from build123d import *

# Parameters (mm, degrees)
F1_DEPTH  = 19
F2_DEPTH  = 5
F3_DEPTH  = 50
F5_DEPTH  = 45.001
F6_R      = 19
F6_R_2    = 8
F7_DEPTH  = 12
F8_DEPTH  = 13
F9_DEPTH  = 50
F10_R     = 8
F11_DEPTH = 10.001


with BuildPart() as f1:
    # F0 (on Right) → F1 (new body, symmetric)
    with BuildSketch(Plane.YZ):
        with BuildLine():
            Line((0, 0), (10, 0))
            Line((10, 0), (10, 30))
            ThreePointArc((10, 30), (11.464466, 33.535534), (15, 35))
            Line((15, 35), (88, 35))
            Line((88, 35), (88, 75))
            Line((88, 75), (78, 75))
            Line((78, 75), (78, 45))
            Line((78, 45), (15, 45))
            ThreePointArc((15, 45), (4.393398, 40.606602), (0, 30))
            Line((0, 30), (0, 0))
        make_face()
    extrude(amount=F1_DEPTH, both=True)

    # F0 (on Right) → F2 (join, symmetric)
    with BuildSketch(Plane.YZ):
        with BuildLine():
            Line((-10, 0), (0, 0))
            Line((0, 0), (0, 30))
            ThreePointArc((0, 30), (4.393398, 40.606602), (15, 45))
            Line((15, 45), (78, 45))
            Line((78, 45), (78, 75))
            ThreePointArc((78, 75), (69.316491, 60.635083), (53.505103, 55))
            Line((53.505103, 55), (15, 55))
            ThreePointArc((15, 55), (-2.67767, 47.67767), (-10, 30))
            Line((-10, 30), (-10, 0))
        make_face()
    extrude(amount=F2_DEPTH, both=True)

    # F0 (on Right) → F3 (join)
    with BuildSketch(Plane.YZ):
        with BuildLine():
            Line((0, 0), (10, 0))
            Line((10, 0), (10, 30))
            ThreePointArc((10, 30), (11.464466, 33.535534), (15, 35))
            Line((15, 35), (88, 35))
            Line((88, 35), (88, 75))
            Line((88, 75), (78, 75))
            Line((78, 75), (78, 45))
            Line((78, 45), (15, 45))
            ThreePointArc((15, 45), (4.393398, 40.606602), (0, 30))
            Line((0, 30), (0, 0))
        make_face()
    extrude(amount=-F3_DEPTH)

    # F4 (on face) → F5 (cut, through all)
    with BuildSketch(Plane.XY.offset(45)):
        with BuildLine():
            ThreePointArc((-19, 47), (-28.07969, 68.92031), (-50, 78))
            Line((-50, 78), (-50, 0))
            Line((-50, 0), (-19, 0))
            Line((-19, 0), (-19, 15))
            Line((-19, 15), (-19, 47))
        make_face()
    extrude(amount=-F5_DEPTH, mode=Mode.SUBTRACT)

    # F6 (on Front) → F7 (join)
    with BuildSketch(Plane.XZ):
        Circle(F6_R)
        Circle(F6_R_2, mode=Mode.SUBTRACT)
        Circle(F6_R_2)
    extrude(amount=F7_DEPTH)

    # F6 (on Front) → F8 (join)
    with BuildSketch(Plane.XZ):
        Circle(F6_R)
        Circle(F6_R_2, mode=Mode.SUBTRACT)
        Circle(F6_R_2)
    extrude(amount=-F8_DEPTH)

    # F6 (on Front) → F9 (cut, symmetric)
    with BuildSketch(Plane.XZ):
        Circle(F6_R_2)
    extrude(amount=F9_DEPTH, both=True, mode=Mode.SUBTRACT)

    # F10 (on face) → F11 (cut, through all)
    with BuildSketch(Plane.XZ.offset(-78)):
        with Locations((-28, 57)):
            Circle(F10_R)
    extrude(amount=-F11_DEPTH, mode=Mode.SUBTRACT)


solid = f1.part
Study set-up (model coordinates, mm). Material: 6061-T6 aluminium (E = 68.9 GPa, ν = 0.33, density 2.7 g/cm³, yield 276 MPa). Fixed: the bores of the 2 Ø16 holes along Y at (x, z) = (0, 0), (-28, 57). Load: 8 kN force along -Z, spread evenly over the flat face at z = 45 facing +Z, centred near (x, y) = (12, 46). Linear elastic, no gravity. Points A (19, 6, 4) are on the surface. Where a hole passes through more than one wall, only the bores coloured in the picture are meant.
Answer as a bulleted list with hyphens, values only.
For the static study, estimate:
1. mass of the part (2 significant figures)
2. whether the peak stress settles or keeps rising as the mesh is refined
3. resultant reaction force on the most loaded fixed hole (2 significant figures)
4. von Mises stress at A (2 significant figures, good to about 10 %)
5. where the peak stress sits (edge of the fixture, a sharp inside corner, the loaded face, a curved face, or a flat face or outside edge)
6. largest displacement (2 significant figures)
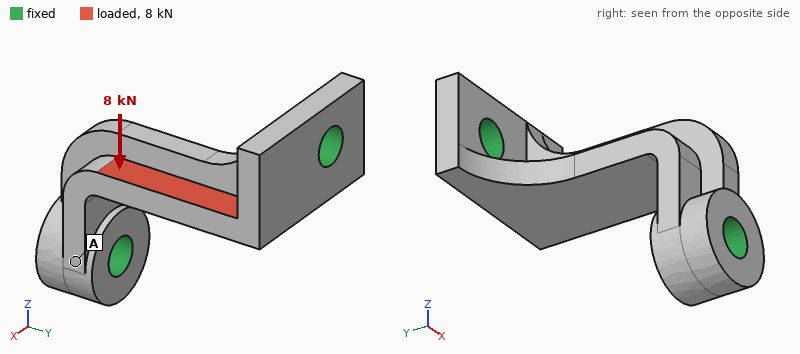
- 270 g
- keeps rising
- 4.2 kN
- 18 MPa
- edge of the fixture
- 0.14 mm
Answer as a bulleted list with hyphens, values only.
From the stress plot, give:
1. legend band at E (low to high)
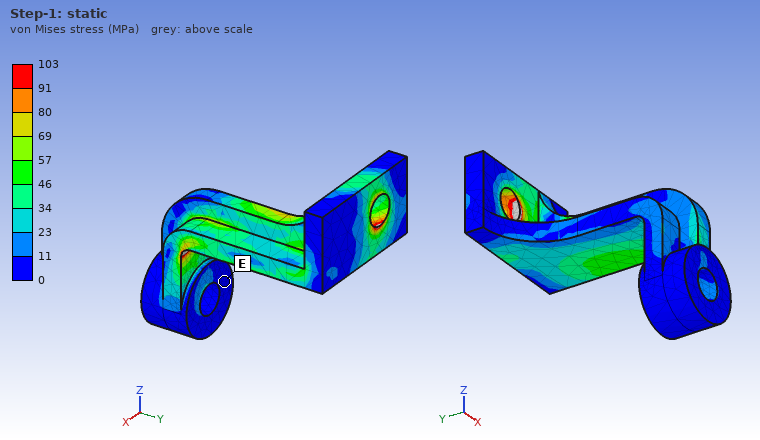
- 0 to 11 MPa
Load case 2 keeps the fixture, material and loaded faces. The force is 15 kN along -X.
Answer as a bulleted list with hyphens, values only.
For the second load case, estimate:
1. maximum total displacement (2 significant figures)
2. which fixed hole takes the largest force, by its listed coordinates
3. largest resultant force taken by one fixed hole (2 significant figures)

- 0.11 mm
- (-28, 57)
- 9.4 kN
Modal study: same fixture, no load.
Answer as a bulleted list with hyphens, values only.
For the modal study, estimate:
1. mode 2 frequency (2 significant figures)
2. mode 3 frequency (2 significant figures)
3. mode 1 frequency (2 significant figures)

- 6500 Hz
- 8100 Hz
- 5300 Hz
